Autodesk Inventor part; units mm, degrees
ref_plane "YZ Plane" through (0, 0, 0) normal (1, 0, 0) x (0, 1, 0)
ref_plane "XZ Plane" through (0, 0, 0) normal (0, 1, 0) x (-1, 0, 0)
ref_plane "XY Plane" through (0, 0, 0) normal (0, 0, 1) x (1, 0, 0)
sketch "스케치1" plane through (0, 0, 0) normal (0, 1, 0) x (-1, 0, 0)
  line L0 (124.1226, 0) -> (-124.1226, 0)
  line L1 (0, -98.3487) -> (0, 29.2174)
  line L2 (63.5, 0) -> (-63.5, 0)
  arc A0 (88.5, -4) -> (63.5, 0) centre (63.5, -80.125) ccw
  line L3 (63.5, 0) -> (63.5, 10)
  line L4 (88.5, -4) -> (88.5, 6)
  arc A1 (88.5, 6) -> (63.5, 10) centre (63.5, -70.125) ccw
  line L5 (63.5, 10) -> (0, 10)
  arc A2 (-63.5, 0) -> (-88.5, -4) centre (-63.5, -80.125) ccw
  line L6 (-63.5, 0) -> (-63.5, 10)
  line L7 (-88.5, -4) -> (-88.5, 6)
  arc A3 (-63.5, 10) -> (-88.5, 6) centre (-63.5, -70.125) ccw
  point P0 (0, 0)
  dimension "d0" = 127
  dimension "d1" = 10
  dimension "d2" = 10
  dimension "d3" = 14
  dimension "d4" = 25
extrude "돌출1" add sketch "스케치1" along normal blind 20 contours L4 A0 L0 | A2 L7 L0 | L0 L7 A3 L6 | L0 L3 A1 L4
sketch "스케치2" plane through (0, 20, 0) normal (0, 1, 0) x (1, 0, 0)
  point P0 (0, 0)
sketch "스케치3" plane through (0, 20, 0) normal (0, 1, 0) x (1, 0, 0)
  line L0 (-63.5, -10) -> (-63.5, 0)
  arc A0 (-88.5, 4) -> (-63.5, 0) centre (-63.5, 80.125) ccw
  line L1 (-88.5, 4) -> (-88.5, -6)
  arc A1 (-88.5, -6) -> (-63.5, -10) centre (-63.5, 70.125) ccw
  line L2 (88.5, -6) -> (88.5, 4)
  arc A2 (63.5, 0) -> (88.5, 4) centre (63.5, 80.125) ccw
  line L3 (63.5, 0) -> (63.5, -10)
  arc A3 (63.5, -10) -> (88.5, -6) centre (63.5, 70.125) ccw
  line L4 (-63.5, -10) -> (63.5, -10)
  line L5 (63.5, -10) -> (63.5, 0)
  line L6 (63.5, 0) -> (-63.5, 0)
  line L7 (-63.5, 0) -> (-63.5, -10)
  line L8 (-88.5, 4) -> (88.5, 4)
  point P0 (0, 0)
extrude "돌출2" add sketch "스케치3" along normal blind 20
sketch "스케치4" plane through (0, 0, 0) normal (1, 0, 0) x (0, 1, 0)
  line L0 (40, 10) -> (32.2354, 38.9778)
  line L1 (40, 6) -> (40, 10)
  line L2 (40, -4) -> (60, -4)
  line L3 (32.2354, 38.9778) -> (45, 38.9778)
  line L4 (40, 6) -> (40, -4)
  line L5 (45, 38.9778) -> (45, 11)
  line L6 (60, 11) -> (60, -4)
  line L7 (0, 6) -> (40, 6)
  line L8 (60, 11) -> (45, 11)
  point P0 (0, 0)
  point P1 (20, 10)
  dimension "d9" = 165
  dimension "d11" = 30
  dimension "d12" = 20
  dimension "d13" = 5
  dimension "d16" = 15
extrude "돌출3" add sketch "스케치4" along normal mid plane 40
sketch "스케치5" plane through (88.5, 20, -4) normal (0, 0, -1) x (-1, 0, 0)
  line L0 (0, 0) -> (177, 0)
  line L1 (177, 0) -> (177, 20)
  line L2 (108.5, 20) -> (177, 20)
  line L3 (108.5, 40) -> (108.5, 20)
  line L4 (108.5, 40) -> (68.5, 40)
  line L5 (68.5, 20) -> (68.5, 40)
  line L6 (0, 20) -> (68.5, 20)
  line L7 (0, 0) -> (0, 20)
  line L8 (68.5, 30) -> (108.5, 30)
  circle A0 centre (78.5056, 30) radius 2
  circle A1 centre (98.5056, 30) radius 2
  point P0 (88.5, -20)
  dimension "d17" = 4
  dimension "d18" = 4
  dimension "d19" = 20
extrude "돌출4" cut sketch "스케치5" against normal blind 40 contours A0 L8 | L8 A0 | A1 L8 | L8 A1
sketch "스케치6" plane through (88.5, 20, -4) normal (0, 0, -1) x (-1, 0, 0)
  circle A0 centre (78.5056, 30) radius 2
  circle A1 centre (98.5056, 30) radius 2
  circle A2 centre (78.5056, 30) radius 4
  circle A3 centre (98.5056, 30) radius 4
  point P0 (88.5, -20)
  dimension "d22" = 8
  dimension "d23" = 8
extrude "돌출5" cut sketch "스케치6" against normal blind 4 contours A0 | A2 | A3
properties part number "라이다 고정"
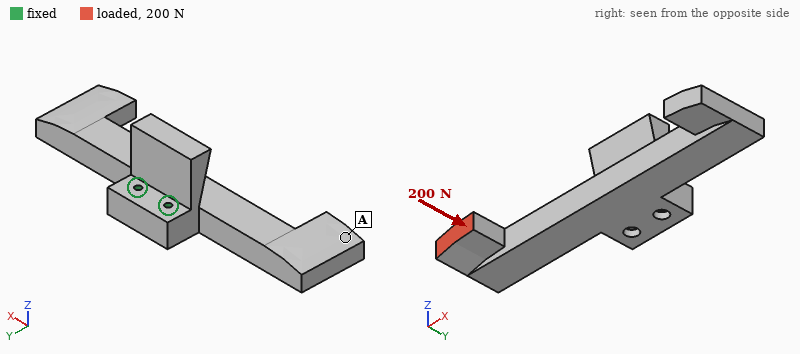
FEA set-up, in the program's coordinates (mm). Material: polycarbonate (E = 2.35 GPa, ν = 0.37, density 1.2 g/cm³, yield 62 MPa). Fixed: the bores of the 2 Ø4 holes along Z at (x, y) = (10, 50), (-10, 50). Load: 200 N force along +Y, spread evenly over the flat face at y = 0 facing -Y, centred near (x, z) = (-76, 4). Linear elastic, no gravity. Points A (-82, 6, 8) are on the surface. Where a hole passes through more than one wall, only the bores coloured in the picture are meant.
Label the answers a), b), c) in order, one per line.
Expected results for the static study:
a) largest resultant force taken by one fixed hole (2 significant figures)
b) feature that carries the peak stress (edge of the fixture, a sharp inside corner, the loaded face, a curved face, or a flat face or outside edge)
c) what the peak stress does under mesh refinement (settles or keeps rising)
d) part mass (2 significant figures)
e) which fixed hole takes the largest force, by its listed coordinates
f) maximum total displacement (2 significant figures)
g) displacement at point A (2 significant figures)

a) 800 N
b) edge of the fixture
c) keeps rising
d) 96 g
e) (-10, 50)
f) 1.5 mm
g) 1.4 mm
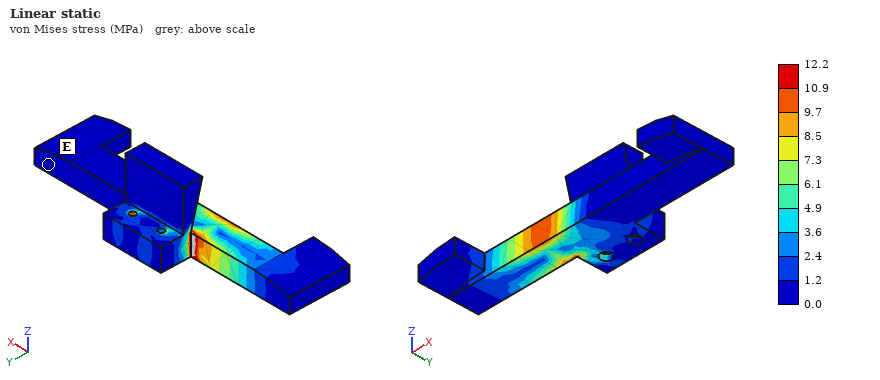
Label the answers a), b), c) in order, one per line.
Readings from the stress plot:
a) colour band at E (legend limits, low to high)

a) 0.0 to 1.2 MPa
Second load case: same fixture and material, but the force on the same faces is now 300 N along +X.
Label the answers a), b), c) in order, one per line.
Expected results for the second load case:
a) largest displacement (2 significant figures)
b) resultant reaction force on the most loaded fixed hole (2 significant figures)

a) 1.8 mm
b) 710 N
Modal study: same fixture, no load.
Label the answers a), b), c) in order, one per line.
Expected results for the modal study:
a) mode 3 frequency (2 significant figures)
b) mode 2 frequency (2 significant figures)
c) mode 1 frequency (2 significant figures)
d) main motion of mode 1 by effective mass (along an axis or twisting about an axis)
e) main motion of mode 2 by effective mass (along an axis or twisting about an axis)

a) 480 Hz
b) 370 Hz
c) 320 Hz
d) twisting about Y
e) along Z
